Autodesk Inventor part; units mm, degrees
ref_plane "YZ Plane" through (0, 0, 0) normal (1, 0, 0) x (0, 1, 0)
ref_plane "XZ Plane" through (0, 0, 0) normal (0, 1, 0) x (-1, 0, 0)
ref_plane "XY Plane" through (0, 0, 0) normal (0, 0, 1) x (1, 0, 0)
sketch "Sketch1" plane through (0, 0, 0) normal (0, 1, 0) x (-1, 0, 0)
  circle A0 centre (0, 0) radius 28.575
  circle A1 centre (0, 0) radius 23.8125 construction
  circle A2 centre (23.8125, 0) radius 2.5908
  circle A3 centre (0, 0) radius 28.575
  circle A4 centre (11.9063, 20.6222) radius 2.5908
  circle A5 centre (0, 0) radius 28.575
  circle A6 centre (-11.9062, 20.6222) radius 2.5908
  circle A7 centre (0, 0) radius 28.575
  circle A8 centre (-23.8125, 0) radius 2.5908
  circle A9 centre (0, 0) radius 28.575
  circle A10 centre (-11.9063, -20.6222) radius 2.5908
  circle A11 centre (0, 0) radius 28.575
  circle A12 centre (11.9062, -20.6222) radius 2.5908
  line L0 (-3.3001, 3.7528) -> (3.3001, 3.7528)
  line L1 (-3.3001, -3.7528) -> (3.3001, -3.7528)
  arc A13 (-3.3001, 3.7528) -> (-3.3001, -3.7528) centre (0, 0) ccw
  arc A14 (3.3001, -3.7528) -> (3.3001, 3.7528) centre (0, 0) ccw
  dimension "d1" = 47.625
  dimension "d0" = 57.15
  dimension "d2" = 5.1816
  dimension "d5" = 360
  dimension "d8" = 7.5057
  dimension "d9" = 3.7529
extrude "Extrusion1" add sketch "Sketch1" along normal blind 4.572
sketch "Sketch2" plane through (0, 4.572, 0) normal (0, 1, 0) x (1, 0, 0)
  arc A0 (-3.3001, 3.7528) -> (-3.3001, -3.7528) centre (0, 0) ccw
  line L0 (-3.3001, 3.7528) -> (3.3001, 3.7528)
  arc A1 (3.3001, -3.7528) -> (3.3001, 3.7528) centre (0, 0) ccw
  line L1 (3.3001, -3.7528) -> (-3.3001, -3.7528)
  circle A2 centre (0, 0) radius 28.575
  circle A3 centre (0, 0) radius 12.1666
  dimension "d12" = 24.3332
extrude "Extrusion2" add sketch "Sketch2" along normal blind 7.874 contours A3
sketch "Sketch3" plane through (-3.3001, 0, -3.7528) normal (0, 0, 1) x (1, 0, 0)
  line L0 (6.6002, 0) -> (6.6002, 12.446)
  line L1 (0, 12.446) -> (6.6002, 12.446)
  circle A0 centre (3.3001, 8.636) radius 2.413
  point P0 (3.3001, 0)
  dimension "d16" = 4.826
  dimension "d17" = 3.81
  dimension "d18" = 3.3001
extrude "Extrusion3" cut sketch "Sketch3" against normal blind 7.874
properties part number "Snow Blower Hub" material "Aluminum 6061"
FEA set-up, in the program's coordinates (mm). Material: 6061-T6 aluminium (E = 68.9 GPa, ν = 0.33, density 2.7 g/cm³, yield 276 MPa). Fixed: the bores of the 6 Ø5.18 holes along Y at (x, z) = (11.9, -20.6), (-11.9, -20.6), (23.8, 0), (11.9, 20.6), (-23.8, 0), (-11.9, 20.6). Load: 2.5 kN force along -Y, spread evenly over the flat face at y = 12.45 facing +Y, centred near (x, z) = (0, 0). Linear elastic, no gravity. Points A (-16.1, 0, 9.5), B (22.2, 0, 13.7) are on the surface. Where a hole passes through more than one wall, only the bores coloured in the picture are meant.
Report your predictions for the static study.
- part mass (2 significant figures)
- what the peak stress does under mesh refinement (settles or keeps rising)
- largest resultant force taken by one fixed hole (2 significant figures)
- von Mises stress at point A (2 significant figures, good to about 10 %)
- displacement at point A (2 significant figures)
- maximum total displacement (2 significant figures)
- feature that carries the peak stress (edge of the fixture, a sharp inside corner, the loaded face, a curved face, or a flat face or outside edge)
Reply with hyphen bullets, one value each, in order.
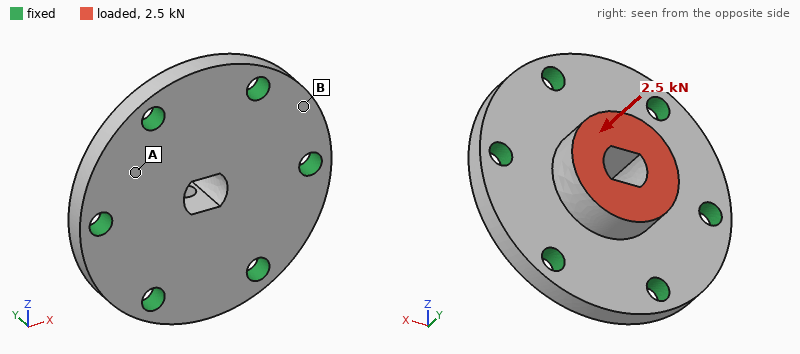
- 37 g
- keeps rising
- 460 N
- 14 MPa
- 5.0 µm
- 15 µm
- edge of the fixture
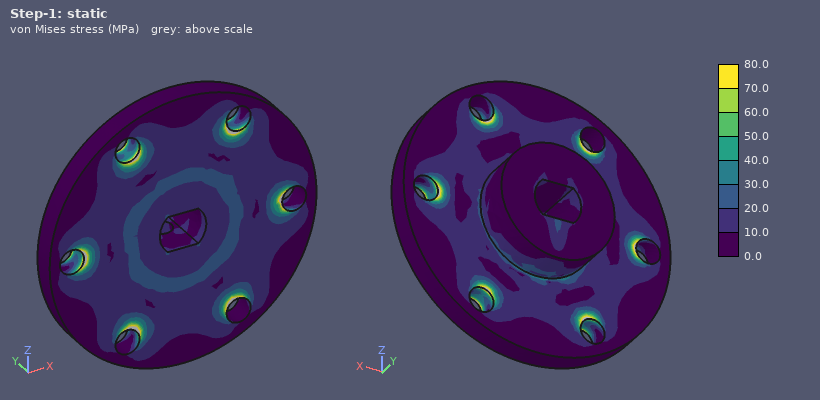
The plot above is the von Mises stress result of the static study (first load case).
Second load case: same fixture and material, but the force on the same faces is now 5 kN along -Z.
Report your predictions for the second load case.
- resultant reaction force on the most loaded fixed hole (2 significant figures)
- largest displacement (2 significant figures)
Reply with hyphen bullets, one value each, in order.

- 1.4 kN
- 33 µm
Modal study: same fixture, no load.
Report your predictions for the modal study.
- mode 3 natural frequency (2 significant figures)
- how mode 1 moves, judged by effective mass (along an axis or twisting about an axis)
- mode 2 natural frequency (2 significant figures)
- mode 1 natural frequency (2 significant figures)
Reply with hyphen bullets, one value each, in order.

- 26 kHz
- along Y
- 26 kHz
- 17 kHz
